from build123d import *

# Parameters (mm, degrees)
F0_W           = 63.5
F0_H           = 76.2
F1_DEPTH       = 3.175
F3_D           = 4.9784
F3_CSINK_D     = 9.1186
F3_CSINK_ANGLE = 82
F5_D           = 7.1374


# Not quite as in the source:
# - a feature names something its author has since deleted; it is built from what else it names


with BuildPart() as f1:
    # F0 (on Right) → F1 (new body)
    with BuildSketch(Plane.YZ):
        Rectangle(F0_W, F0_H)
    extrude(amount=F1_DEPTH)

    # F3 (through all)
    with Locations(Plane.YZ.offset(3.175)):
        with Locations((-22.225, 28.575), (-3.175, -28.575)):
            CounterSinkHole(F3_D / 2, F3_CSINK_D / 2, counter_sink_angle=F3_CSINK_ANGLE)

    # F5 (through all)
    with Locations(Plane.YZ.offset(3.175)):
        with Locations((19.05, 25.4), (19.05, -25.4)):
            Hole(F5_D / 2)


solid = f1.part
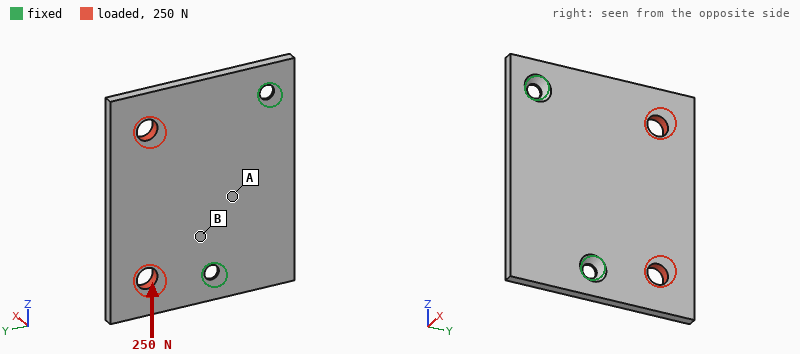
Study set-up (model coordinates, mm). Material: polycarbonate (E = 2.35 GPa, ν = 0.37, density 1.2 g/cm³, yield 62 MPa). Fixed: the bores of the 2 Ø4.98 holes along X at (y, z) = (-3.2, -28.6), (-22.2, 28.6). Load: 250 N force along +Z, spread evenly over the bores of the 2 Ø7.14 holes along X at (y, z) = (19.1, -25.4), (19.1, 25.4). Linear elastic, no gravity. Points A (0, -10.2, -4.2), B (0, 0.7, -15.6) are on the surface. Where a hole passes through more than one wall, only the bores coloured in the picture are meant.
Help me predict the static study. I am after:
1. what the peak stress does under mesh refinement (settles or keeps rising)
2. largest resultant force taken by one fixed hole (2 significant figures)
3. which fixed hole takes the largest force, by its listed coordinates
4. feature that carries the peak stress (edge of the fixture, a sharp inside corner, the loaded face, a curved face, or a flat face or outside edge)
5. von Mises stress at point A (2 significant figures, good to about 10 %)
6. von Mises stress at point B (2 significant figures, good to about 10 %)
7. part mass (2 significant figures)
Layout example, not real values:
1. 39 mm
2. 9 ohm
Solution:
1. keeps rising
2. 210 N
3. (-3.2, -28.6)
4. edge of the fixture
5. 1.7 MPa
6. 3.6 MPa
7. 18 g
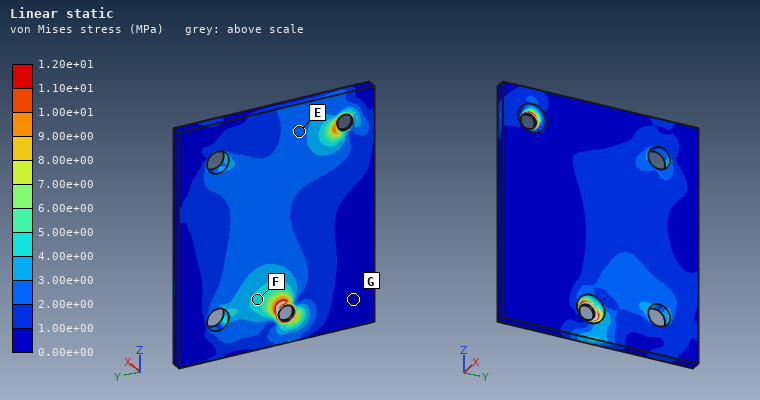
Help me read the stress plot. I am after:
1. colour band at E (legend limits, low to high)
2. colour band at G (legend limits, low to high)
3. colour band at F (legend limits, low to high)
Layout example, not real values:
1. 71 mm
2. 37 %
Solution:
1. 2.00e+00 to 3.00e+00 MPa
2. 0.00e+00 to 1.00e+00 MPa
3. 4.00e+00 to 5.00e+00 MPa
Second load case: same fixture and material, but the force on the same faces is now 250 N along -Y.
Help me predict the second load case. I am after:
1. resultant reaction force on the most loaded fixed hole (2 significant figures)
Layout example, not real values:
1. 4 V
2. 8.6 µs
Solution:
1. 130 N
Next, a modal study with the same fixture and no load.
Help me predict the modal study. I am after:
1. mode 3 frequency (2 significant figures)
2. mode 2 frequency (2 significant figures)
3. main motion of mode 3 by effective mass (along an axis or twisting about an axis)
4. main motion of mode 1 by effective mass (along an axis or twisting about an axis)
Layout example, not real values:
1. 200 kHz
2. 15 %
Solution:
1. 750 Hz
2. 580 Hz
3. along X
4. along X
